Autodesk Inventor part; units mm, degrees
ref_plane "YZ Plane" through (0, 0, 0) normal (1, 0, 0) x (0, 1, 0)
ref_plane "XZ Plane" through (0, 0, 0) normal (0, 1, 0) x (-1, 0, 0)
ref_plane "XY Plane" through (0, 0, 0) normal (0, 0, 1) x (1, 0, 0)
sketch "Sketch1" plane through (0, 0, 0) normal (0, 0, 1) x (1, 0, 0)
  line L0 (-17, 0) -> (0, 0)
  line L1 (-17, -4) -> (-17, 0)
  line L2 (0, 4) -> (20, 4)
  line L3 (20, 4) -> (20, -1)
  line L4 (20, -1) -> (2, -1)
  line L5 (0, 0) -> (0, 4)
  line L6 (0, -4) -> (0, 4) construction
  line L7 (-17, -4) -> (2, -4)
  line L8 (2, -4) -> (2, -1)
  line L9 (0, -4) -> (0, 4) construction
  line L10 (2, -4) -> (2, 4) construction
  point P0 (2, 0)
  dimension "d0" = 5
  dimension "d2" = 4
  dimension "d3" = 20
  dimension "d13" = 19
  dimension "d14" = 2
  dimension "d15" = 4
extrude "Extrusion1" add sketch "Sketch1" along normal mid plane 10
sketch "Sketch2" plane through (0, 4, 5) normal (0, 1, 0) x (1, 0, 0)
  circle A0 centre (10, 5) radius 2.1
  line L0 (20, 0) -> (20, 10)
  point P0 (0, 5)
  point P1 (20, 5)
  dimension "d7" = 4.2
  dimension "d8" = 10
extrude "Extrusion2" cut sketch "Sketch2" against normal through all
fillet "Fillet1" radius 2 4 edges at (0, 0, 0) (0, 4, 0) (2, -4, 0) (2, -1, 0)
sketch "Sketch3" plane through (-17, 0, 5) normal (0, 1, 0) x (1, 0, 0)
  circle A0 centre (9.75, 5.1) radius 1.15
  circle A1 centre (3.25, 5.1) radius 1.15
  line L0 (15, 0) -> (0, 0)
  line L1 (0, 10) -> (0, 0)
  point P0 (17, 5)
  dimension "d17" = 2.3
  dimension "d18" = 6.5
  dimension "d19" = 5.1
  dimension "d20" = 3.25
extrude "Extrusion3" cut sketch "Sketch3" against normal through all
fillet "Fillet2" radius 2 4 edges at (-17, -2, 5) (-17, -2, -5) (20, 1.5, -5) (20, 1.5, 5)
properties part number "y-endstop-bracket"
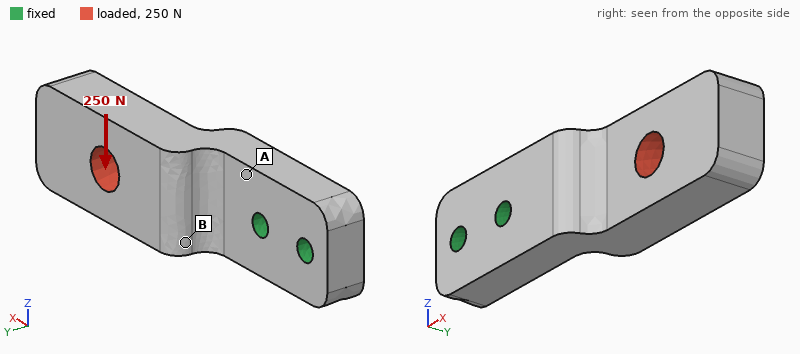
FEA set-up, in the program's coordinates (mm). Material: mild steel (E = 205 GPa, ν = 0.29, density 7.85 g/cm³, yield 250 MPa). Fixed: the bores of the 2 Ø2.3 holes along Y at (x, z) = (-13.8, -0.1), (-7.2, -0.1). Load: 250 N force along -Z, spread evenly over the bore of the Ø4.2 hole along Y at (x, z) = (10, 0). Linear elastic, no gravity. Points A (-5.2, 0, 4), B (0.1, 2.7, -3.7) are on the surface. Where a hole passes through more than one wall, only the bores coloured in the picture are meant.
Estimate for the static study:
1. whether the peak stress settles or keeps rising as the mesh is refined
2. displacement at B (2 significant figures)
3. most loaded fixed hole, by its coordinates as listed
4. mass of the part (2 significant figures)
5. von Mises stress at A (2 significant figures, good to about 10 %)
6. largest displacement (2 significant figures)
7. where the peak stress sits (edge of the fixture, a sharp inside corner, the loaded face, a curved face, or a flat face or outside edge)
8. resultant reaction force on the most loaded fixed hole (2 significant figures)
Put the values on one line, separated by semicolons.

keeps rising; 6.2 µm; (-7.2, -0.1); 13 g; 46 MPa; 24 µm; edge of the fixture; 640 N
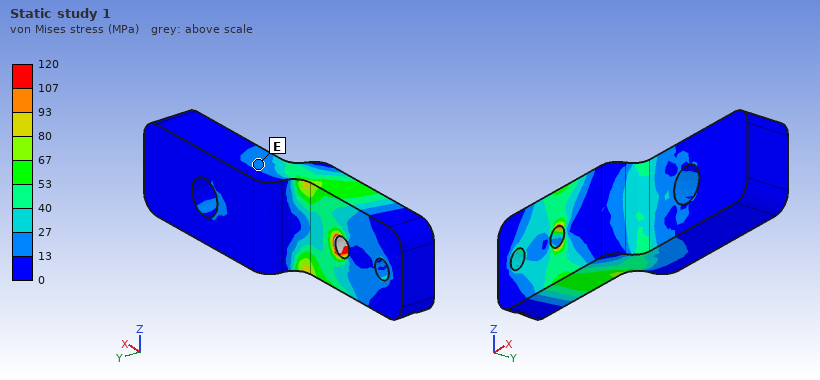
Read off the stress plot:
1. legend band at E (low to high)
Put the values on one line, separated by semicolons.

13 to 27 MPa
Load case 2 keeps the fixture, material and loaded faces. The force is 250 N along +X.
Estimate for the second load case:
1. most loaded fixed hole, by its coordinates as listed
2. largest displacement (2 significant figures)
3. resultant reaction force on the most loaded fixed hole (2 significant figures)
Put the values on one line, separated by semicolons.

(-7.2, -0.1); 17 µm; 210 N
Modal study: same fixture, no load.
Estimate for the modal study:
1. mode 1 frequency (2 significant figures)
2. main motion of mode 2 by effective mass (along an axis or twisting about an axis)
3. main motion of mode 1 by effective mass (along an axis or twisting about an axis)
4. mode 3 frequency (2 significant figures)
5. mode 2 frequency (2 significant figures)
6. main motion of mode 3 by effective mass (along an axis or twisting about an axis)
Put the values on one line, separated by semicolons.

4000 Hz; along Z; along Y; 17 kHz; 7200 Hz; twisting about X
